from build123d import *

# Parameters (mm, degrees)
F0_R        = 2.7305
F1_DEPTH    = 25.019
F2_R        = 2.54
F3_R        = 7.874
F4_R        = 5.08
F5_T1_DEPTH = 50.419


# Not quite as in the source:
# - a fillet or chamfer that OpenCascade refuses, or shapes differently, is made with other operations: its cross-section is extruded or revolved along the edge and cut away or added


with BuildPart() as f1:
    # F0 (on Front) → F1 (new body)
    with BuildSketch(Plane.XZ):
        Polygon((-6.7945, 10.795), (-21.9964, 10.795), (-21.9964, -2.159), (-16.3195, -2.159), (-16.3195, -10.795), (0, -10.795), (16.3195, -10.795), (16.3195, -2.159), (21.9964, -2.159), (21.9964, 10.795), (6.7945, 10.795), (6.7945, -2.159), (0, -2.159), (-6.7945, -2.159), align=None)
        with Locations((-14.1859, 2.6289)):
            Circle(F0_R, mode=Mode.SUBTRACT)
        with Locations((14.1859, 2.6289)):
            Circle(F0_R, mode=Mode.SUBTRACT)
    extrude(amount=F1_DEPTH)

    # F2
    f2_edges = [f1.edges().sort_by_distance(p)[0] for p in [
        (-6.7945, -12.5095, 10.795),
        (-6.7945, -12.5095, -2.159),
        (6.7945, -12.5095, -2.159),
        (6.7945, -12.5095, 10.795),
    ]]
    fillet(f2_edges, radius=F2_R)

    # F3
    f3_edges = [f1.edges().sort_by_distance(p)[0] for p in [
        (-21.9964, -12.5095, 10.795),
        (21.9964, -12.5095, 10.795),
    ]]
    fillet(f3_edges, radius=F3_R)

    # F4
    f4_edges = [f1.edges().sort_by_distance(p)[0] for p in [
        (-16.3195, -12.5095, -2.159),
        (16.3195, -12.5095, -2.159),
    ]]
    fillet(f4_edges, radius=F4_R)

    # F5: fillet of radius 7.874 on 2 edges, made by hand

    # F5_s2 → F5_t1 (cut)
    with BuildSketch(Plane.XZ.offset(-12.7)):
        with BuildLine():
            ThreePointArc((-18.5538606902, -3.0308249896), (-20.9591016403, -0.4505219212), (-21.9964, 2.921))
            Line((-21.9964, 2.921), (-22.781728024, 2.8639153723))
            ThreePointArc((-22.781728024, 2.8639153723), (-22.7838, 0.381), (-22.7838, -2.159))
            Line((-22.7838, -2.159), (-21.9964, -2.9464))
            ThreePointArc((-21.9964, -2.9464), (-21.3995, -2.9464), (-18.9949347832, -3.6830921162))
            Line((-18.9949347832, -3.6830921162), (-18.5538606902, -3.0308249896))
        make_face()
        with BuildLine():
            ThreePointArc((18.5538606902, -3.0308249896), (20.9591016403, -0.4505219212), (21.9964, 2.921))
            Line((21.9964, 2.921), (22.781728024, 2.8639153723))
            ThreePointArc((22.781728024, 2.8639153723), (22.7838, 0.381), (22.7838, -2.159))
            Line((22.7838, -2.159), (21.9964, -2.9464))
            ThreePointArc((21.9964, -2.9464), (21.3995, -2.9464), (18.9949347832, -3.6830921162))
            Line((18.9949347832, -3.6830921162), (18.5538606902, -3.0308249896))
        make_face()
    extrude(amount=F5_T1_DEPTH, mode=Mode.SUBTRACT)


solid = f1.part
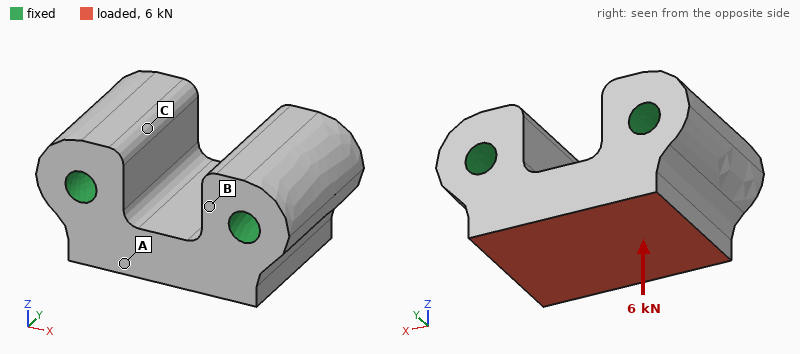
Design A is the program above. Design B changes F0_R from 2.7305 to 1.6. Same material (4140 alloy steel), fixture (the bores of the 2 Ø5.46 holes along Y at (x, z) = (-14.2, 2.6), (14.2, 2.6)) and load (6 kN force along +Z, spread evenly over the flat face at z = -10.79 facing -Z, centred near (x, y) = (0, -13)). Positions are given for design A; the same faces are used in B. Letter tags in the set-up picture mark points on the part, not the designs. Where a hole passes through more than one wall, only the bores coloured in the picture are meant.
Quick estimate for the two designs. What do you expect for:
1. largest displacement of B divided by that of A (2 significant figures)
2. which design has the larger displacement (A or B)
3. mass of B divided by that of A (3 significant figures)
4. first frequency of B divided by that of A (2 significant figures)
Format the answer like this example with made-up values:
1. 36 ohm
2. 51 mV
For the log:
1. 1.1
2. B
3. 1.05
4. 0.86
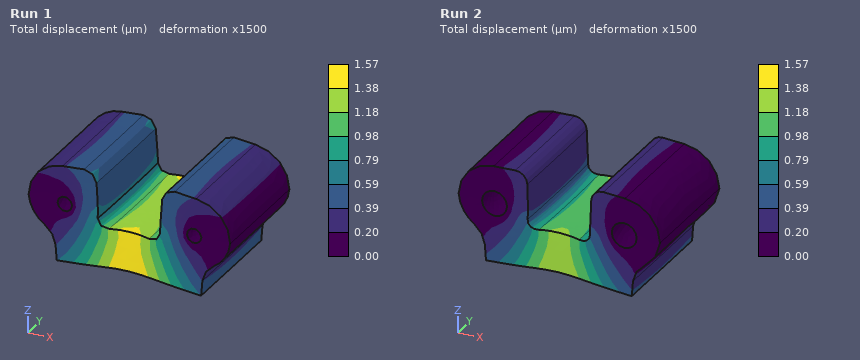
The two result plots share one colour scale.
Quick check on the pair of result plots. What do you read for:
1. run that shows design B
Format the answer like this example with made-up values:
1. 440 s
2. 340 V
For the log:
1. Run 1
